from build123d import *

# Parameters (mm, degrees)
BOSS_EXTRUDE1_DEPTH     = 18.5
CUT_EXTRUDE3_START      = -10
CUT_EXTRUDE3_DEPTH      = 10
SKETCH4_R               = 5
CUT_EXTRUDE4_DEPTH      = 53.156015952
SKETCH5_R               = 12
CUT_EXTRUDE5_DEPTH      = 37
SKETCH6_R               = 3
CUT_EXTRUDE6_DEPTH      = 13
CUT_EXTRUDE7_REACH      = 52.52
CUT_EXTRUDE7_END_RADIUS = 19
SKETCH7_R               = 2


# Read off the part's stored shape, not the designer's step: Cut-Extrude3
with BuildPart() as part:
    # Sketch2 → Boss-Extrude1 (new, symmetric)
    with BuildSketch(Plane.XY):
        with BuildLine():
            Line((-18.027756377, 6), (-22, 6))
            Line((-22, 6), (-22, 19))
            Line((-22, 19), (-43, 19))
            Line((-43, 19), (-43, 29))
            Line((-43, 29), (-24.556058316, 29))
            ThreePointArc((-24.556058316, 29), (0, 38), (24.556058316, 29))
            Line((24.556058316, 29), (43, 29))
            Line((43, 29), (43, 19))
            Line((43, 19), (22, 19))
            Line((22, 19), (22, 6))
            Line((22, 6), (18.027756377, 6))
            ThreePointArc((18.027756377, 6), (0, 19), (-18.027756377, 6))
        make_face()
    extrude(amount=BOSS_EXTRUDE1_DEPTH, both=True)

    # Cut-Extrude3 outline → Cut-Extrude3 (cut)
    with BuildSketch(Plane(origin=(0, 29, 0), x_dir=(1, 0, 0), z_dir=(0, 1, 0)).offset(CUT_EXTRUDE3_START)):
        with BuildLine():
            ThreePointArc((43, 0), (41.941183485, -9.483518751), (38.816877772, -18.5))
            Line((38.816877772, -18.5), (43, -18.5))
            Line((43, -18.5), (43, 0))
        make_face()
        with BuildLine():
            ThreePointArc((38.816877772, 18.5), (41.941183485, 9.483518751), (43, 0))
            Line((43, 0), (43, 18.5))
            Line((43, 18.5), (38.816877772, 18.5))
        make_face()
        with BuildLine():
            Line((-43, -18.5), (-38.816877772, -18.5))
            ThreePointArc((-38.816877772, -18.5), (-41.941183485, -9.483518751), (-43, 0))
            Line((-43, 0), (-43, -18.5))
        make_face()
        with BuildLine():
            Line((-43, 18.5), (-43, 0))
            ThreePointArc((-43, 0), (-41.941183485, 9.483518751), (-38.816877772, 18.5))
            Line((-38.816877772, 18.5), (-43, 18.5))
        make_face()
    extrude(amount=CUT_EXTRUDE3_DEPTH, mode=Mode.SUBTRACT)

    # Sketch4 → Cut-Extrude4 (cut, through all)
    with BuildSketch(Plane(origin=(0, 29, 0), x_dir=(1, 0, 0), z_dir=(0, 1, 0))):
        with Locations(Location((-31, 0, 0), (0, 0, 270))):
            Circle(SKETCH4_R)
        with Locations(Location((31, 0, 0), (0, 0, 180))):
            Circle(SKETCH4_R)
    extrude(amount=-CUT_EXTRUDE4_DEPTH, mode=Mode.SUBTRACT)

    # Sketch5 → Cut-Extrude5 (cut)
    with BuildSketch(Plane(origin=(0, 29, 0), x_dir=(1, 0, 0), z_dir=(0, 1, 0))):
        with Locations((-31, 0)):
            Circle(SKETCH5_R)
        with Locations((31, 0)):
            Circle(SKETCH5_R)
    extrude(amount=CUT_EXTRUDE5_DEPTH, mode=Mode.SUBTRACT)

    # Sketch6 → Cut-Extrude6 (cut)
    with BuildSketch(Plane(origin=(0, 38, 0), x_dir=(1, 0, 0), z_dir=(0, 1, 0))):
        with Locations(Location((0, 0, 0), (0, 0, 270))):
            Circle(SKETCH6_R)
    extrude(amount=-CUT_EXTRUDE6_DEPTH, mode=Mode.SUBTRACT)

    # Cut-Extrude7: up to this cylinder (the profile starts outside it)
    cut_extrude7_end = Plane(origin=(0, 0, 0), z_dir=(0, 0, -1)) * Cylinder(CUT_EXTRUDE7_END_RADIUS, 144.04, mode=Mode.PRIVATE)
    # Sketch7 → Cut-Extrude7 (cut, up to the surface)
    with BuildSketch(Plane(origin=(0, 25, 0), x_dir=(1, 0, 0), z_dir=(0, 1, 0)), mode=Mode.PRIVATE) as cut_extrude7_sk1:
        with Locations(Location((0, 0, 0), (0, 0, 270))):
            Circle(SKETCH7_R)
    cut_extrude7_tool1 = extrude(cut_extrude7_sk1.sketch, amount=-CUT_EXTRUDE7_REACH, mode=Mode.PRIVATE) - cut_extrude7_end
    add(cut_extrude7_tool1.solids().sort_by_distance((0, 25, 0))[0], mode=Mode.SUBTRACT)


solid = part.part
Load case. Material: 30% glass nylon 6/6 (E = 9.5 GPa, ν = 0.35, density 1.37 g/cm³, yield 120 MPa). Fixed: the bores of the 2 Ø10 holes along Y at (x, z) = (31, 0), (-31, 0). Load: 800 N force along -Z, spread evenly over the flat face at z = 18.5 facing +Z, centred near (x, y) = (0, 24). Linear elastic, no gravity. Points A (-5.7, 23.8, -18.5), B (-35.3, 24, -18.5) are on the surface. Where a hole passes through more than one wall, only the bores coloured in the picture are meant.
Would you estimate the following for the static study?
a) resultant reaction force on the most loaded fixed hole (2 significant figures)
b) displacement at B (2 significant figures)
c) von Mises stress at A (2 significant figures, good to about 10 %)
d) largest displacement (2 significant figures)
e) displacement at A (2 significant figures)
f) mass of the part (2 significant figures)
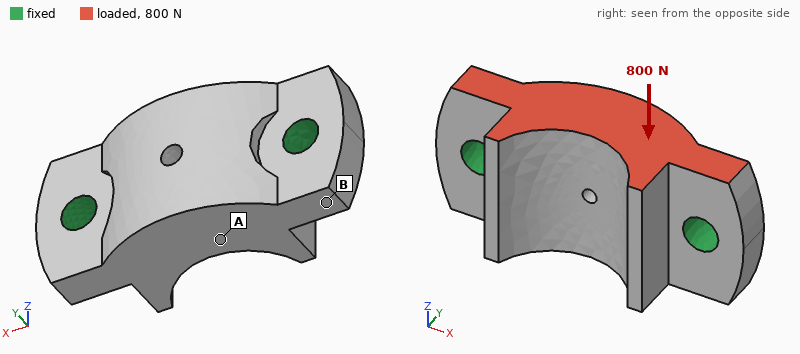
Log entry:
400 N
1.9 µm
1.1 MPa
8.2 µm
4.9 µm
66 g
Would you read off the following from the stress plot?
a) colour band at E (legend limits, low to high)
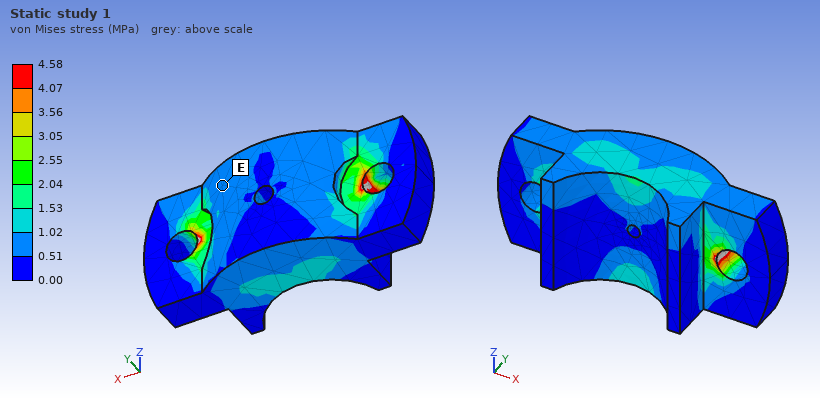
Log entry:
0.51 to 1.02 MPa
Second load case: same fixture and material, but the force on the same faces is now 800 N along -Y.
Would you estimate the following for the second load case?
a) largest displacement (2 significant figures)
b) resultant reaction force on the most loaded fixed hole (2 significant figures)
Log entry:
47 µm
410 N
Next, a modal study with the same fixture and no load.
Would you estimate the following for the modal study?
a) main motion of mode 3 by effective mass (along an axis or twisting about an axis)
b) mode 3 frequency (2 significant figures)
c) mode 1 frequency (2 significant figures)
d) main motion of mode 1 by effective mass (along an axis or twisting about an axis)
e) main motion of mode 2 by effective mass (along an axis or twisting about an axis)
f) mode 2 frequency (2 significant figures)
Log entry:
along Z
8000 Hz
5100 Hz
twisting about X
along Y
6200 Hz
